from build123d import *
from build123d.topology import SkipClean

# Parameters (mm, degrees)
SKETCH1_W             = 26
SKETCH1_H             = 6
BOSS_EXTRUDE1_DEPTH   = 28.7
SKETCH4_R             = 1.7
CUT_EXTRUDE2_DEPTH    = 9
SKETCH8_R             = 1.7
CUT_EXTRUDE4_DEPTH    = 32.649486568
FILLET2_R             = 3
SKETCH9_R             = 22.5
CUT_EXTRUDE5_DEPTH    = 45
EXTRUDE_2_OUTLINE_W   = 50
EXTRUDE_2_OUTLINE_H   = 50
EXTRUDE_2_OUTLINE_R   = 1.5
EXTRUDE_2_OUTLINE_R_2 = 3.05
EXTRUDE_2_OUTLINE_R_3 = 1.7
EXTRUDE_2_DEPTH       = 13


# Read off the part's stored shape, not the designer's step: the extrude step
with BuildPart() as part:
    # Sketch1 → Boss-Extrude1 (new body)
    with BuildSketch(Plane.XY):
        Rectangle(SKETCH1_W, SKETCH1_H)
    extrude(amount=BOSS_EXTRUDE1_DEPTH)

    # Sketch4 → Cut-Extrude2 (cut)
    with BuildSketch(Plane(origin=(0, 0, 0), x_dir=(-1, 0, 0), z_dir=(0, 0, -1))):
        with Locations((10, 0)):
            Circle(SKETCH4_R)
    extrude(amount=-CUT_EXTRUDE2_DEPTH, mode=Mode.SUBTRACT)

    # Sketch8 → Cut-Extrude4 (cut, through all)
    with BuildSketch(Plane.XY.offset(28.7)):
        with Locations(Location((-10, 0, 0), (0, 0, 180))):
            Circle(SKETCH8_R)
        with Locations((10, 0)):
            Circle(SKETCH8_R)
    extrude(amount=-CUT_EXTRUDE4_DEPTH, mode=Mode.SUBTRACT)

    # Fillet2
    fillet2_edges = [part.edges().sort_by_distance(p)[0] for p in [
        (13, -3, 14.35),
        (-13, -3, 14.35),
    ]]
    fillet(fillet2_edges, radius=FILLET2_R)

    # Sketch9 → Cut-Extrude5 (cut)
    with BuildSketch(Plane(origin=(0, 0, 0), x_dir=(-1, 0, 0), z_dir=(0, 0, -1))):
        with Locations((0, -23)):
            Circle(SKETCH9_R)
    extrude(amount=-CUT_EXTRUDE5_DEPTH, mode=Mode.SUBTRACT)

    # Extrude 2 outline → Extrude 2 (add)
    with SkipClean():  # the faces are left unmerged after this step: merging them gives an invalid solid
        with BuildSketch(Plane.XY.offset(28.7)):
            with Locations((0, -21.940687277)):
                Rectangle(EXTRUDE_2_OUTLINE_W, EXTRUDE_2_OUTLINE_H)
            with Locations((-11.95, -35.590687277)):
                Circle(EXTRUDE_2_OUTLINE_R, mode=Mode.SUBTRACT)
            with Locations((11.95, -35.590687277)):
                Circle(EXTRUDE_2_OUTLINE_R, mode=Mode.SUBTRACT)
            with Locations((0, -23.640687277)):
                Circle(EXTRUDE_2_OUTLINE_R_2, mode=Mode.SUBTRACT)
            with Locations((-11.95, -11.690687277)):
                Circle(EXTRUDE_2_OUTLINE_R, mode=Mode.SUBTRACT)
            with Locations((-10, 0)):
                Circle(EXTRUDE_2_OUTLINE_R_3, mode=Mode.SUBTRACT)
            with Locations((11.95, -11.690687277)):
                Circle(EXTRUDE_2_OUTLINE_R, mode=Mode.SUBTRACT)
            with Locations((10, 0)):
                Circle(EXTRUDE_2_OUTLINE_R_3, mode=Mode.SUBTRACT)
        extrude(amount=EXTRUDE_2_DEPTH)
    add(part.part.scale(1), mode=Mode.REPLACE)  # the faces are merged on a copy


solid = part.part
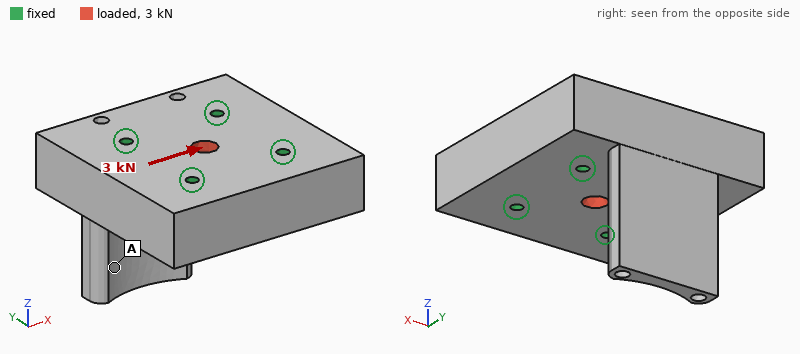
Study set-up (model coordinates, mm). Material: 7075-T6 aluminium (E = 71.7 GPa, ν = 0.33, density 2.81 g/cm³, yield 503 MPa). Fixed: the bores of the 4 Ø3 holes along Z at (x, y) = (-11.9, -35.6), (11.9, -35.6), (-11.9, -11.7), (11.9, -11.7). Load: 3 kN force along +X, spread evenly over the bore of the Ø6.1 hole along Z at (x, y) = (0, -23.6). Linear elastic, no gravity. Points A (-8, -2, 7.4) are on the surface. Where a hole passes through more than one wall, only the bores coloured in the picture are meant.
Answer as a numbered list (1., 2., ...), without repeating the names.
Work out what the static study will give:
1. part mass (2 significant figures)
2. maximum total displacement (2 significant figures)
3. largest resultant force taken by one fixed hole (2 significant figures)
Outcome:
1. 97 g
2. 1.9 µm
3. 790 N
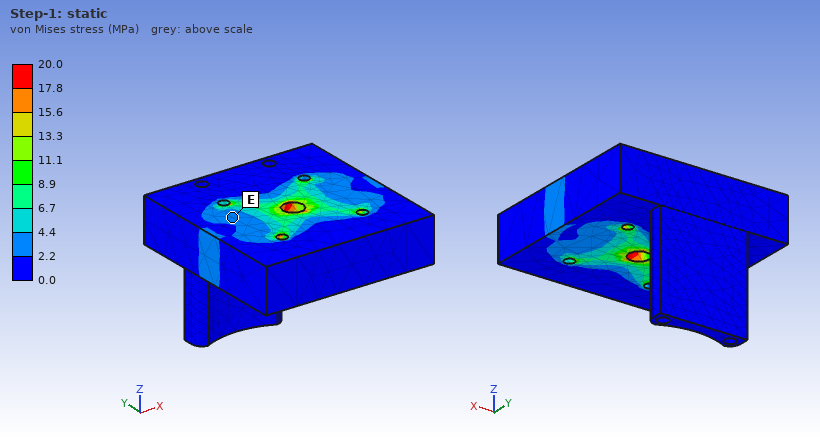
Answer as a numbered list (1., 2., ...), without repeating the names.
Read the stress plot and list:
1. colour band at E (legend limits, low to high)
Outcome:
1. 2.2 to 4.4 MPa
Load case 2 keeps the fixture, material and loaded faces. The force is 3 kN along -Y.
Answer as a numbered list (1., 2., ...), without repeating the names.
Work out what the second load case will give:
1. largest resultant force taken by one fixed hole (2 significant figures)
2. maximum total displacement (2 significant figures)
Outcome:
1. 790 N
2. 1.9 µm
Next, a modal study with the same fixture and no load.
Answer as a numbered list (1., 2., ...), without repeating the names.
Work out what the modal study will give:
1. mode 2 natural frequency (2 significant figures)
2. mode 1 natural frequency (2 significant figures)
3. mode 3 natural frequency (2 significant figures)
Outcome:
1. 9900 Hz
2. 4200 Hz
3. 12 kHz
